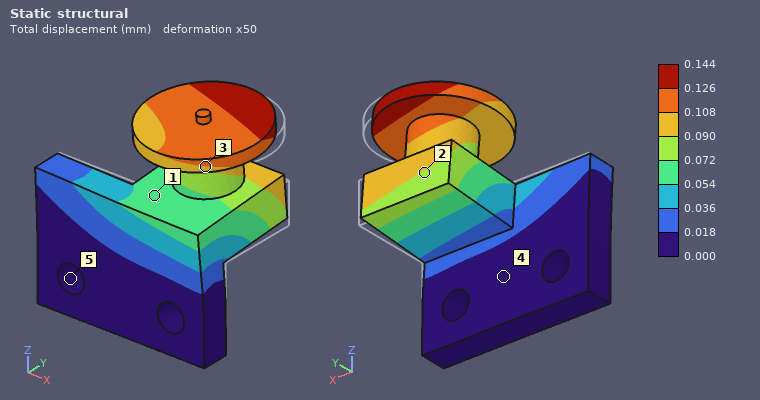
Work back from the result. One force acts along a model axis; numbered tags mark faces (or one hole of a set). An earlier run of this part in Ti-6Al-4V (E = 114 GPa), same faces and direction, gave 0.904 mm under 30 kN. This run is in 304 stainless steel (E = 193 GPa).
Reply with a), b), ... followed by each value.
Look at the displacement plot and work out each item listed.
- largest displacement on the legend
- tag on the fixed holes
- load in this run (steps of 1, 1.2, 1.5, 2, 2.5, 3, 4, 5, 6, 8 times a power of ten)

a) 0.144 mm
b) 5
c) 8 kN
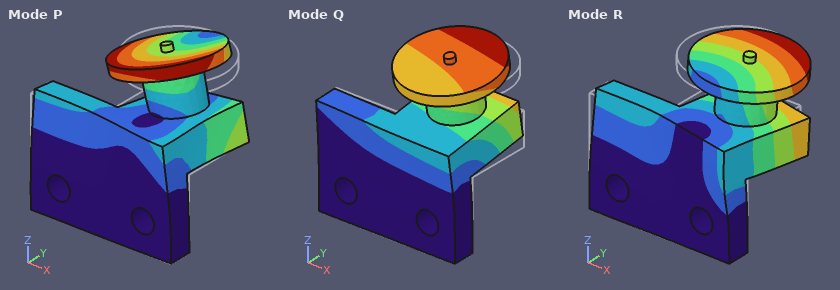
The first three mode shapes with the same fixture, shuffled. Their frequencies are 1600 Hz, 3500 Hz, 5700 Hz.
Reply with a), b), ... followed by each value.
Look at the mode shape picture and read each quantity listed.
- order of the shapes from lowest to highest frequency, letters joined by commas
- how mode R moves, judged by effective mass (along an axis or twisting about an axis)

a) Q, R, P
b) along X
